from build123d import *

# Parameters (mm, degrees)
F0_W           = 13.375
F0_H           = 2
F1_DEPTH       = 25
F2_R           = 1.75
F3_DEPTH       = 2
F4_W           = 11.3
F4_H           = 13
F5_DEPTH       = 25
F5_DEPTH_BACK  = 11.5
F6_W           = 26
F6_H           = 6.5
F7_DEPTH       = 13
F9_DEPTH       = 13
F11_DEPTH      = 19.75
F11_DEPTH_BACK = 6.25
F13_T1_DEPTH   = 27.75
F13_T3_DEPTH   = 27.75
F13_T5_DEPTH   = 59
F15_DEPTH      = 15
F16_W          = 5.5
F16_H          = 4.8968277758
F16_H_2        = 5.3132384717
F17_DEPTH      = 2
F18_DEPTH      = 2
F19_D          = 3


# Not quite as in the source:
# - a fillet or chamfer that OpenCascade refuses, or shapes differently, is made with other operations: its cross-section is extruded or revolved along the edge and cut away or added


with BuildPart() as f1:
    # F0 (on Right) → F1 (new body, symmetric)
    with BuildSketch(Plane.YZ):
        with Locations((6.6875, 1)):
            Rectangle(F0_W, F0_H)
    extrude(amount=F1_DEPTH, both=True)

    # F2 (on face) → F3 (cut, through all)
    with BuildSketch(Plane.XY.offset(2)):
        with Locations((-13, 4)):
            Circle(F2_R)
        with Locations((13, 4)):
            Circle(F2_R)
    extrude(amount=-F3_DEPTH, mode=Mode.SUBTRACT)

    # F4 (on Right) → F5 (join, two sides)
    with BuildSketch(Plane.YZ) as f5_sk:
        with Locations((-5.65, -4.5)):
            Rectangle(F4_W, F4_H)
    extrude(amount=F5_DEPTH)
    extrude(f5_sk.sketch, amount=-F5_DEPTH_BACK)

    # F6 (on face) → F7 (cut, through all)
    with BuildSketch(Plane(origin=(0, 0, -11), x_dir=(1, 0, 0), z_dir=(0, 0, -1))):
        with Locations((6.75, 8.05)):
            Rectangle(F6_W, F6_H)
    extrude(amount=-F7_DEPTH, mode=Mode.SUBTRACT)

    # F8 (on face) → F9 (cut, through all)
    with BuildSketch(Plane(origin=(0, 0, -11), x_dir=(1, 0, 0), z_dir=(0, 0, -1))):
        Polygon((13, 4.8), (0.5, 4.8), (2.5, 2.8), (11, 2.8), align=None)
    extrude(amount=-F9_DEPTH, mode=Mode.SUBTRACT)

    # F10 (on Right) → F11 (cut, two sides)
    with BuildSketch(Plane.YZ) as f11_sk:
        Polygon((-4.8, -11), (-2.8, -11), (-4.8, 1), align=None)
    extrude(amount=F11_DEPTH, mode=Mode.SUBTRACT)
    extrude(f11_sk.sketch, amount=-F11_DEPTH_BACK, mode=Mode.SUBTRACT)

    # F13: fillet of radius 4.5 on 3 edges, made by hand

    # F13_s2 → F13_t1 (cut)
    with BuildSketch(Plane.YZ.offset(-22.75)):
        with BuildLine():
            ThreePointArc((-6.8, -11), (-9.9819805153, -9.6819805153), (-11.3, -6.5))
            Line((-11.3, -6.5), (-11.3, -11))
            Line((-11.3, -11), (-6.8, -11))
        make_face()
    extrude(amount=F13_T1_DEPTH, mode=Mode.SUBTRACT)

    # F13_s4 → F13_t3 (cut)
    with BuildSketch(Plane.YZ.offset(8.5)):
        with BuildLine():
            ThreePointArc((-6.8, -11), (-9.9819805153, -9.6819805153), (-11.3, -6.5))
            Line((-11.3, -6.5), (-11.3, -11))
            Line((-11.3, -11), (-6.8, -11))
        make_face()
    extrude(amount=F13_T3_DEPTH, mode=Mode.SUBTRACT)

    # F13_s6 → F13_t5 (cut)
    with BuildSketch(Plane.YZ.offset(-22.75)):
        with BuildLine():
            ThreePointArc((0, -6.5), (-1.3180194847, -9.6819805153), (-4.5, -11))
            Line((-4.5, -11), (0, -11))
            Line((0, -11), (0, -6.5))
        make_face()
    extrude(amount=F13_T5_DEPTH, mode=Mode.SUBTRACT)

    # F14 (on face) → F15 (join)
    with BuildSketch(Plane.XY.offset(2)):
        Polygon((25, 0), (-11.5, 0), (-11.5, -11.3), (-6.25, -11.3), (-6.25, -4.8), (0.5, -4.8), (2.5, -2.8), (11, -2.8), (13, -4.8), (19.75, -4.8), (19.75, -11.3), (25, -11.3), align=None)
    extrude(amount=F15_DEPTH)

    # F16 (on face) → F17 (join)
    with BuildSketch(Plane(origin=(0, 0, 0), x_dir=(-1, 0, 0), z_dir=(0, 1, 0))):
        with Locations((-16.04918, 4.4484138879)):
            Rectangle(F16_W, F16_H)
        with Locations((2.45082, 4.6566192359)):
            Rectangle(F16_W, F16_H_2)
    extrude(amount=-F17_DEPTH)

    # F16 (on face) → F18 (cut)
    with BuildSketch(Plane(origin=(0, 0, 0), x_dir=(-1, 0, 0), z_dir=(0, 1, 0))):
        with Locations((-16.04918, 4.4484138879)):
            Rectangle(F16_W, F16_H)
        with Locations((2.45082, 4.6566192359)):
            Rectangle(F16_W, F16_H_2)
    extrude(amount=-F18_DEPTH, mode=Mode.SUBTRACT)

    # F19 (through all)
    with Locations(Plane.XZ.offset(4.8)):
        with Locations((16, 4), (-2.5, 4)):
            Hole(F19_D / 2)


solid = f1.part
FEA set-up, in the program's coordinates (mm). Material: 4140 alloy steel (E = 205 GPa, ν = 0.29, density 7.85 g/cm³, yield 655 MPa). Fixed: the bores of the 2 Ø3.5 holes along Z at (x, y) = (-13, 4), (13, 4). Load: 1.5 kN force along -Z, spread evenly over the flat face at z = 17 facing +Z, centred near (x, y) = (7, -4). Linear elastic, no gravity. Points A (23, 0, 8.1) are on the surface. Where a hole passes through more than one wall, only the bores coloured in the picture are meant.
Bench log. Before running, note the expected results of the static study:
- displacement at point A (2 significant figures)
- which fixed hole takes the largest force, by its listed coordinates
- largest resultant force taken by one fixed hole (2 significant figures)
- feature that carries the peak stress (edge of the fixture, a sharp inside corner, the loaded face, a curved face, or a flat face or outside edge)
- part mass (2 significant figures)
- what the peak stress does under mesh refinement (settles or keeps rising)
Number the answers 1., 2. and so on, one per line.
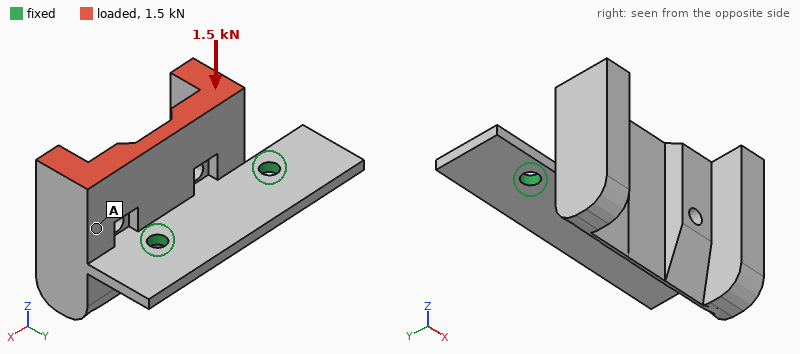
1. 0.063 mm
2. (13, 4)
3. 1.1 kN
4. edge of the fixture
5. 55 g
6. keeps rising
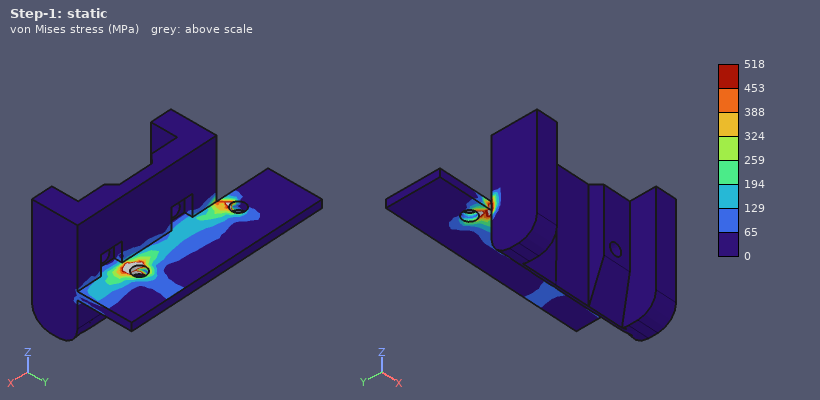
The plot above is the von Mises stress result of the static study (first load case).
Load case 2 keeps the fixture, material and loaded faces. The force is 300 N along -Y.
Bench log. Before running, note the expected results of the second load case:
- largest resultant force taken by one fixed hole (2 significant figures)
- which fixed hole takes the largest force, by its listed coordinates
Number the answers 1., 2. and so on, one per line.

1. 220 N
2. (13, 4)
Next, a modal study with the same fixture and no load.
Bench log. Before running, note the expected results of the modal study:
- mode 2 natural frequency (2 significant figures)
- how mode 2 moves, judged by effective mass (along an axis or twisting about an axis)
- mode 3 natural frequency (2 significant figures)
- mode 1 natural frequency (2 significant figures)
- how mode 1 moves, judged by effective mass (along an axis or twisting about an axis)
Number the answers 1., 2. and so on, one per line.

1. 5600 Hz
2. twisting about Y
3. 9400 Hz
4. 2200 Hz
5. along Z
